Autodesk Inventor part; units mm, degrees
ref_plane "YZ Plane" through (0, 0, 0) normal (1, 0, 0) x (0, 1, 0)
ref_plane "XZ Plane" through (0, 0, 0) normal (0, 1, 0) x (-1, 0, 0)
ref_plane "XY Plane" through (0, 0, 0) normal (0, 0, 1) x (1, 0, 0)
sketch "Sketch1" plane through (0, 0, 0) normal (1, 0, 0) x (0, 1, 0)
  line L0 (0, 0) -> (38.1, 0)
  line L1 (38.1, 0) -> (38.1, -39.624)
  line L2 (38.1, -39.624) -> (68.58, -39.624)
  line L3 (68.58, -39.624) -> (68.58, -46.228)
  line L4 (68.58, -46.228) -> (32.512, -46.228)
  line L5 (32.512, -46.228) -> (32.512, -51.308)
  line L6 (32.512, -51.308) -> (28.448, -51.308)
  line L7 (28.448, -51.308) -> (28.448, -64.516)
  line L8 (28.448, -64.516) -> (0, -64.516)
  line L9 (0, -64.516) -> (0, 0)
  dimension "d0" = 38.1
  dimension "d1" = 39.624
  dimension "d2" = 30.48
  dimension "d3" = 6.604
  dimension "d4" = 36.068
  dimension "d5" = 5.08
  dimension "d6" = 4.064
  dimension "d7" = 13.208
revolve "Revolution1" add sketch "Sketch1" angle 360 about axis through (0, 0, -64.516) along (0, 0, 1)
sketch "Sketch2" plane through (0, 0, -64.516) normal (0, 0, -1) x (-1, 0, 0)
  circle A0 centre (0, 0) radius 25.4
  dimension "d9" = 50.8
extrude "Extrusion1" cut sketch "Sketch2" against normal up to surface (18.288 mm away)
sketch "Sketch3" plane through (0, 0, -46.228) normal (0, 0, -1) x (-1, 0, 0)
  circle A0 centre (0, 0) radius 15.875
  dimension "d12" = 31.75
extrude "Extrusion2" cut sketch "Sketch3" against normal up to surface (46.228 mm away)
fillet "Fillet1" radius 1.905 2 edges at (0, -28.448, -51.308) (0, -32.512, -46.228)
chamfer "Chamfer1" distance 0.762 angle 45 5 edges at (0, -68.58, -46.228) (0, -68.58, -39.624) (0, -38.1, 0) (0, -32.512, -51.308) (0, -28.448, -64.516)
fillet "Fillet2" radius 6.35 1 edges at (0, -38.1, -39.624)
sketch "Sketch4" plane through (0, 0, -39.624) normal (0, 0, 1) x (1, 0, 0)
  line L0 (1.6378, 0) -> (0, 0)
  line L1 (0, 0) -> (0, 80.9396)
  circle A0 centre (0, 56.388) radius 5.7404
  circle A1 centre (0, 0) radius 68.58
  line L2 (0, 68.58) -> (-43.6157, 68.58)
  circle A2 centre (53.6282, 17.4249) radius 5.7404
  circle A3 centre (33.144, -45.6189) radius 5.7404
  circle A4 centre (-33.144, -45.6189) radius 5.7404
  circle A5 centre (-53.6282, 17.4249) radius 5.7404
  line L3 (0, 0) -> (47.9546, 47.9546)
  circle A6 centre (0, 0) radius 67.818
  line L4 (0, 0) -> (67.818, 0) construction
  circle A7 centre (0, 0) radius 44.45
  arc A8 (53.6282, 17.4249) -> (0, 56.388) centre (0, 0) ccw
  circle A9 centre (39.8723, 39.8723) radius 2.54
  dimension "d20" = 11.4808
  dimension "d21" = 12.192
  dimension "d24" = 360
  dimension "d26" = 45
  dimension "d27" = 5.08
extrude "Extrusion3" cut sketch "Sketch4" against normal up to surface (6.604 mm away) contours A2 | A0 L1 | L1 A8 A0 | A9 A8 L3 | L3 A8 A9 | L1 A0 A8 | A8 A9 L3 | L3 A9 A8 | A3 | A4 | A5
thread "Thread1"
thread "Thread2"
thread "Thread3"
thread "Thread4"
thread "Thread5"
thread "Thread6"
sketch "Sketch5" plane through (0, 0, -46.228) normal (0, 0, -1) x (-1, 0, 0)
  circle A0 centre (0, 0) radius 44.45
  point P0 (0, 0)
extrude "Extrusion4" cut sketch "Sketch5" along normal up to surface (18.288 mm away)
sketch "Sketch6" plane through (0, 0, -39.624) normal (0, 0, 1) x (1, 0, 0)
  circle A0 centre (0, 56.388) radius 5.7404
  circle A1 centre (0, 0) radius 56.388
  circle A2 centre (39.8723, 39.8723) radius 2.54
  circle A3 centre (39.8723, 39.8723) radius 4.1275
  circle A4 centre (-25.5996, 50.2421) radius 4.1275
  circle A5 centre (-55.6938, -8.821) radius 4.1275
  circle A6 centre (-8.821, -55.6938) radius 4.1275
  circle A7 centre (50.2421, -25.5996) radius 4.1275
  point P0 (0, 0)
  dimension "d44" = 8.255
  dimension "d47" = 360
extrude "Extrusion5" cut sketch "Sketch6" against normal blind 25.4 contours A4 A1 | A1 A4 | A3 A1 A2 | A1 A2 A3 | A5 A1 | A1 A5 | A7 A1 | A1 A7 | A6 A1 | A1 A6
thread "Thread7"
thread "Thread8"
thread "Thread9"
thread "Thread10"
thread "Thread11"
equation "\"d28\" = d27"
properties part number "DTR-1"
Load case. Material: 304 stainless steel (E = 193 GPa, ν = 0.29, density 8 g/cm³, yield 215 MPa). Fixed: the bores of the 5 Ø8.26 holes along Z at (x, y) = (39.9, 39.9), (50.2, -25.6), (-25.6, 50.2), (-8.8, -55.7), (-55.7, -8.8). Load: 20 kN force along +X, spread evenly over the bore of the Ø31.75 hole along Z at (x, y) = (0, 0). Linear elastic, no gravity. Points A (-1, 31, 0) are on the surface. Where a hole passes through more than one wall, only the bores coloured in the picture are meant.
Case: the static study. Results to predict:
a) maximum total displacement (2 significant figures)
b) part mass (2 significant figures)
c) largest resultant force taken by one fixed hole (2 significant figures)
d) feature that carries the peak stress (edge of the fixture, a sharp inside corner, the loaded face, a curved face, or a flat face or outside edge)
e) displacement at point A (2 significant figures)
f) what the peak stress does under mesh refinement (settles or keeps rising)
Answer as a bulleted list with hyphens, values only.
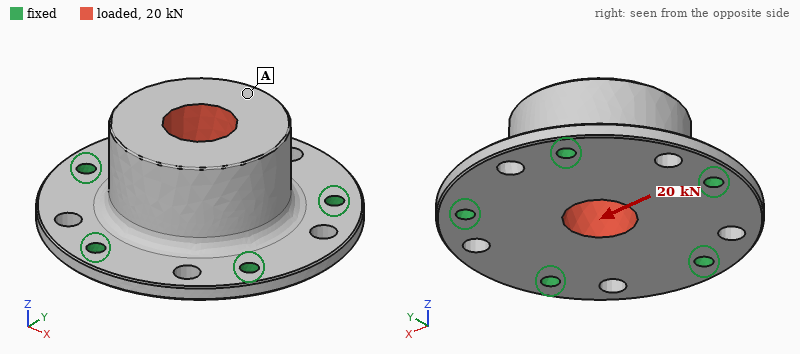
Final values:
- 20 µm
- 1.9 kg
- 6.4 kN
- edge of the fixture
- 16 µm
- keeps rising
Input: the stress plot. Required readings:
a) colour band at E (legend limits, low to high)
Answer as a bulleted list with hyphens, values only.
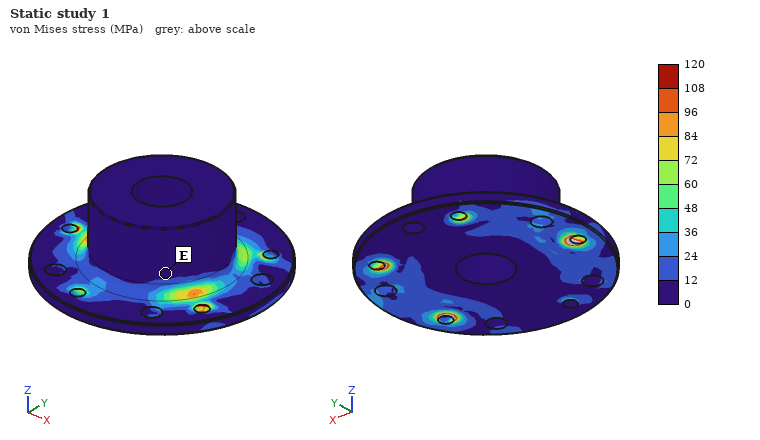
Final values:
- 0 to 12 MPa
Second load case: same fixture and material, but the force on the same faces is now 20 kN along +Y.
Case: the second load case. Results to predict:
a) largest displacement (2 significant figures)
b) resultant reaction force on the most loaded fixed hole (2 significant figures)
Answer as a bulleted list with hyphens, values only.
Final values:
- 20 µm
- 6.4 kN
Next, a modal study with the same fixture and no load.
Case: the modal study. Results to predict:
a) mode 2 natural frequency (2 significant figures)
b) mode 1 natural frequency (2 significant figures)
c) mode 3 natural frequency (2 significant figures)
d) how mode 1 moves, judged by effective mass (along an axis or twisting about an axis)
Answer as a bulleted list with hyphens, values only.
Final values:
- 4400 Hz
- 4100 Hz
- 4400 Hz
- along Z
